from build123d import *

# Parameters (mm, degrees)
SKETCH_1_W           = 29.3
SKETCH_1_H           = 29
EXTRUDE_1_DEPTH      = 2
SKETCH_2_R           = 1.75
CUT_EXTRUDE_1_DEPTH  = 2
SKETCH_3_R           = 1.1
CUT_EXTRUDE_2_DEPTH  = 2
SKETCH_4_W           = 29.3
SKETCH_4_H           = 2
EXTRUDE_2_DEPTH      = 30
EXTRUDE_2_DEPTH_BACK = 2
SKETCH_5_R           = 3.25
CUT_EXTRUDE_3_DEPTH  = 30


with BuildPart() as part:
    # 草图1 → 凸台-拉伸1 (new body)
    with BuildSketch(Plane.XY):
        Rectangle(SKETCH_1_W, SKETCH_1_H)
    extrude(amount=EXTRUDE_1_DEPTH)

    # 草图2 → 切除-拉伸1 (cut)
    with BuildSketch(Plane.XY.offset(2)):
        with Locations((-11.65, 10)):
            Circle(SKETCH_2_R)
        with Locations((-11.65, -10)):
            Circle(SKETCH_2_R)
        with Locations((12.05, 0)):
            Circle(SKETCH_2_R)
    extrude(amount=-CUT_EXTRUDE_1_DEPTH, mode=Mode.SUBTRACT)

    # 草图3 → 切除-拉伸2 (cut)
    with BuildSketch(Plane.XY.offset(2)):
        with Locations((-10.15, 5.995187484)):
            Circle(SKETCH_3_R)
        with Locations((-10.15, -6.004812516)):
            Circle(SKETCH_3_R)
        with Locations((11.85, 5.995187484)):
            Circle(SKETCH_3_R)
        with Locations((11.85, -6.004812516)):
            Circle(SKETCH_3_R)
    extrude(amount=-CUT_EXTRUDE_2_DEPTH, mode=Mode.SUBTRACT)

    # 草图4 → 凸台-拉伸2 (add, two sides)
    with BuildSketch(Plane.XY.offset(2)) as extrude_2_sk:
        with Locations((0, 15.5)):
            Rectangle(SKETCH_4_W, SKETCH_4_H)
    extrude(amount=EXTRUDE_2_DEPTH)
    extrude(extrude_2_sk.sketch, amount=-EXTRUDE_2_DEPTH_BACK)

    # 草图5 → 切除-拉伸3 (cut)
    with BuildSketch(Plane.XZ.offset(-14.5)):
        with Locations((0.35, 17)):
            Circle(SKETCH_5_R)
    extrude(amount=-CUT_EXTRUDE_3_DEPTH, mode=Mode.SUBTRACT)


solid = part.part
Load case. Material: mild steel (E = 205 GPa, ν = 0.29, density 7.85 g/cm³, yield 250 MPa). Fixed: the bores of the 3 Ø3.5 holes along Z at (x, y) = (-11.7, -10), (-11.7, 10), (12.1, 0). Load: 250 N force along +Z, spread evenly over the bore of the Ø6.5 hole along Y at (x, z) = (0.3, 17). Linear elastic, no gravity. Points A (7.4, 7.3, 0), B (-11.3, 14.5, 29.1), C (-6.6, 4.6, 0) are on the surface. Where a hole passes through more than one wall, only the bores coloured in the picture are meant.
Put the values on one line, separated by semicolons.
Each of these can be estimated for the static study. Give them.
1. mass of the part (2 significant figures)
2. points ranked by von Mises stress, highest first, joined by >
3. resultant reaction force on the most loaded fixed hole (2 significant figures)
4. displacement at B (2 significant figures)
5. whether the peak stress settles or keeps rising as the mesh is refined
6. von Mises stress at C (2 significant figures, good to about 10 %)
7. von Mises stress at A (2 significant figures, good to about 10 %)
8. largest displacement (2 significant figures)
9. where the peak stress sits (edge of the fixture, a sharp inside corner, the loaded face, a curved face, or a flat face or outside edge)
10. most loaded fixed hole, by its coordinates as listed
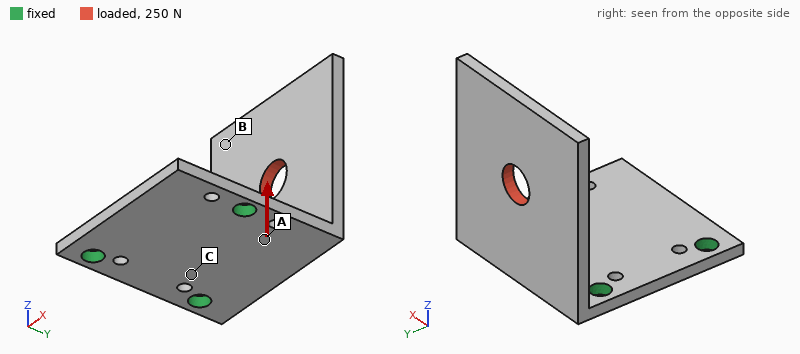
27 g; A > C > B; 190 N; 0.078 mm; keeps rising; 31 MPa; 64 MPa; 0.11 mm; edge of the fixture; (-11.7, 10)
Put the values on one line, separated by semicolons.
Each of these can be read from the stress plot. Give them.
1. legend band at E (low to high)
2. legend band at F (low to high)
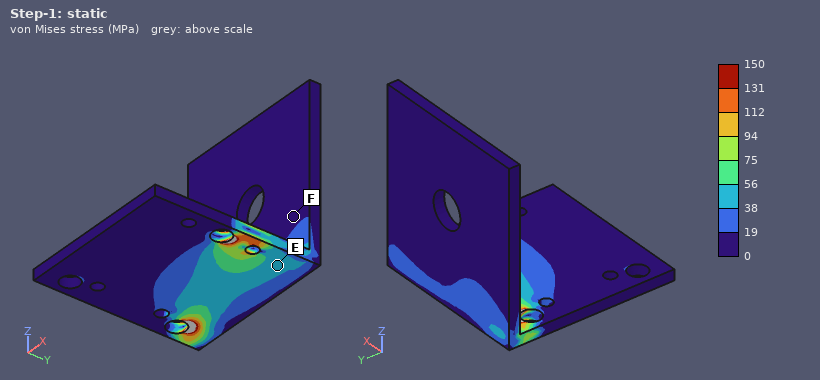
38 to 56 MPa; 0 to 19 MPa
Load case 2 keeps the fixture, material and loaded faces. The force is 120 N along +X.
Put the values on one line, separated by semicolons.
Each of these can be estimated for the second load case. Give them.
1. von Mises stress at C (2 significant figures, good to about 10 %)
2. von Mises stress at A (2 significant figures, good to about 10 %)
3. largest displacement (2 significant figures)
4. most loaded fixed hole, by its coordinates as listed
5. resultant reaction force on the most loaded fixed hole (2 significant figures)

16 MPa; 37 MPa; 60 µm; (-11.7, 10); 110 N
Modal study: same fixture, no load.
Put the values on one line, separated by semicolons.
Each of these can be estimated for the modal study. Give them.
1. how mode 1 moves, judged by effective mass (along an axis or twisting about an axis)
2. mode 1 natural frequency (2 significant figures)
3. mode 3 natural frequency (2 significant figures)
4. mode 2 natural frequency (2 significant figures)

along Y; 1200 Hz; 4100 Hz; 2700 Hz
